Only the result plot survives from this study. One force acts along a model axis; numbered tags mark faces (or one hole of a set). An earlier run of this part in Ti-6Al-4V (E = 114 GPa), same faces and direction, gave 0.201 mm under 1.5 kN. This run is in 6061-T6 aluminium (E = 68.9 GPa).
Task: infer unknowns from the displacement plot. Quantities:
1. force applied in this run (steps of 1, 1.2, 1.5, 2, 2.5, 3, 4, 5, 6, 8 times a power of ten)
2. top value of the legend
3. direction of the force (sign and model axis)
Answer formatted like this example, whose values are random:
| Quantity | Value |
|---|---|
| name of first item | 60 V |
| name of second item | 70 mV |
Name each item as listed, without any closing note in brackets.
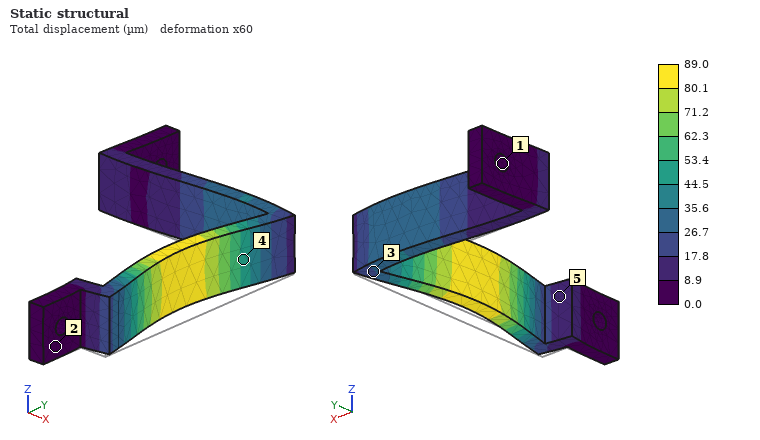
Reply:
| Quantity | Value |
|---|---|
| force applied in this run | 400 N |
| top value of the legend | 89.0 µm |
| direction of the force | -X |
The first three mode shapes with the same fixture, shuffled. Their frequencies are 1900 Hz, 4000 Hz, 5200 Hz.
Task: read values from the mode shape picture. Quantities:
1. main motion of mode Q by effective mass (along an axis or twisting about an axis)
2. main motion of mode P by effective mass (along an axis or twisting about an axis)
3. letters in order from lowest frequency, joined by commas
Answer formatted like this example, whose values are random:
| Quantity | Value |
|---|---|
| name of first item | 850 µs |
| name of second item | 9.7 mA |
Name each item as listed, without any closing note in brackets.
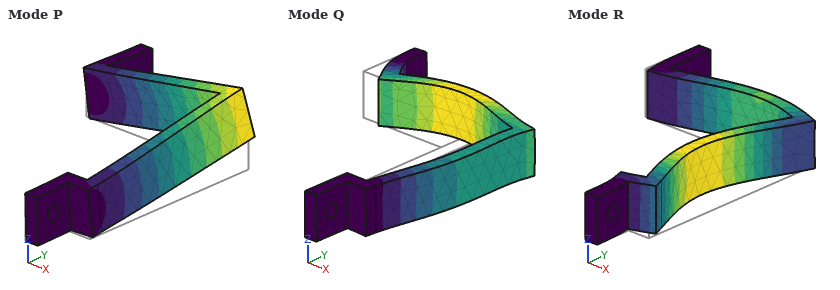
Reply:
| Quantity | Value |
|---|---|
| main motion of mode Q by effective mass | along X |
| main motion of mode P by effective mass | along Z |
| letters in order from lowest frequency, joined by commas | P, R, Q |
